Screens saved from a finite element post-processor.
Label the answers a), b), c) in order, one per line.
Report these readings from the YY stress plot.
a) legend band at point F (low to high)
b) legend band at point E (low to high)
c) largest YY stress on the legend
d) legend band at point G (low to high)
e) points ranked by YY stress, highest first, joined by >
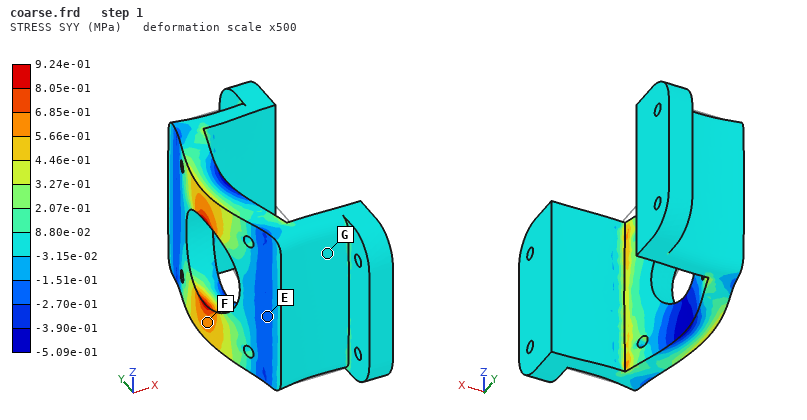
a) 5.66e-01 to 6.85e-01 MPa
b) -2.70e-01 to -1.51e-01 MPa
c) 9.24e-01 MPa
d) -3.15e-02 to 8.80e-02 MPa
e) F > G > E
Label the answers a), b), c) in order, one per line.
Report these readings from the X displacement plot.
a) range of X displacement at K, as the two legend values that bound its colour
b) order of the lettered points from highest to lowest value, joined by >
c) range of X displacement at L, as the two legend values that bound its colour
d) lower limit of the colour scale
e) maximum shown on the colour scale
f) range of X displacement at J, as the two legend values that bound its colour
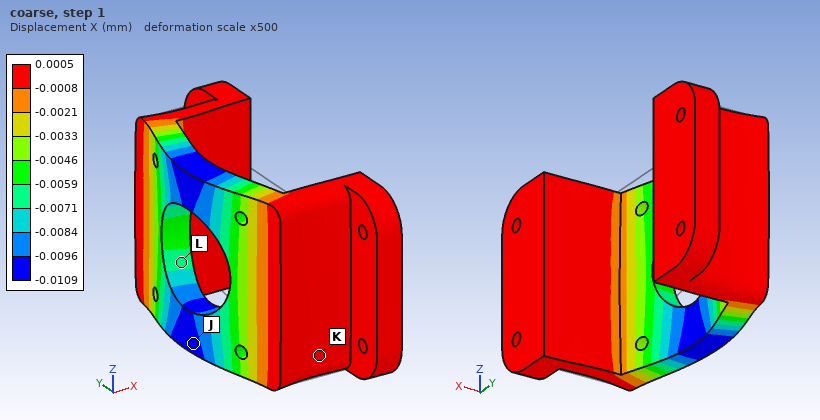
a) -0.0008 to 0.0005 mm
b) K > L > J
c) -0.0071 to -0.0059 mm
d) -0.0109 mm
e) 0.0005 mm
f) -0.0109 to -0.0096 mm
